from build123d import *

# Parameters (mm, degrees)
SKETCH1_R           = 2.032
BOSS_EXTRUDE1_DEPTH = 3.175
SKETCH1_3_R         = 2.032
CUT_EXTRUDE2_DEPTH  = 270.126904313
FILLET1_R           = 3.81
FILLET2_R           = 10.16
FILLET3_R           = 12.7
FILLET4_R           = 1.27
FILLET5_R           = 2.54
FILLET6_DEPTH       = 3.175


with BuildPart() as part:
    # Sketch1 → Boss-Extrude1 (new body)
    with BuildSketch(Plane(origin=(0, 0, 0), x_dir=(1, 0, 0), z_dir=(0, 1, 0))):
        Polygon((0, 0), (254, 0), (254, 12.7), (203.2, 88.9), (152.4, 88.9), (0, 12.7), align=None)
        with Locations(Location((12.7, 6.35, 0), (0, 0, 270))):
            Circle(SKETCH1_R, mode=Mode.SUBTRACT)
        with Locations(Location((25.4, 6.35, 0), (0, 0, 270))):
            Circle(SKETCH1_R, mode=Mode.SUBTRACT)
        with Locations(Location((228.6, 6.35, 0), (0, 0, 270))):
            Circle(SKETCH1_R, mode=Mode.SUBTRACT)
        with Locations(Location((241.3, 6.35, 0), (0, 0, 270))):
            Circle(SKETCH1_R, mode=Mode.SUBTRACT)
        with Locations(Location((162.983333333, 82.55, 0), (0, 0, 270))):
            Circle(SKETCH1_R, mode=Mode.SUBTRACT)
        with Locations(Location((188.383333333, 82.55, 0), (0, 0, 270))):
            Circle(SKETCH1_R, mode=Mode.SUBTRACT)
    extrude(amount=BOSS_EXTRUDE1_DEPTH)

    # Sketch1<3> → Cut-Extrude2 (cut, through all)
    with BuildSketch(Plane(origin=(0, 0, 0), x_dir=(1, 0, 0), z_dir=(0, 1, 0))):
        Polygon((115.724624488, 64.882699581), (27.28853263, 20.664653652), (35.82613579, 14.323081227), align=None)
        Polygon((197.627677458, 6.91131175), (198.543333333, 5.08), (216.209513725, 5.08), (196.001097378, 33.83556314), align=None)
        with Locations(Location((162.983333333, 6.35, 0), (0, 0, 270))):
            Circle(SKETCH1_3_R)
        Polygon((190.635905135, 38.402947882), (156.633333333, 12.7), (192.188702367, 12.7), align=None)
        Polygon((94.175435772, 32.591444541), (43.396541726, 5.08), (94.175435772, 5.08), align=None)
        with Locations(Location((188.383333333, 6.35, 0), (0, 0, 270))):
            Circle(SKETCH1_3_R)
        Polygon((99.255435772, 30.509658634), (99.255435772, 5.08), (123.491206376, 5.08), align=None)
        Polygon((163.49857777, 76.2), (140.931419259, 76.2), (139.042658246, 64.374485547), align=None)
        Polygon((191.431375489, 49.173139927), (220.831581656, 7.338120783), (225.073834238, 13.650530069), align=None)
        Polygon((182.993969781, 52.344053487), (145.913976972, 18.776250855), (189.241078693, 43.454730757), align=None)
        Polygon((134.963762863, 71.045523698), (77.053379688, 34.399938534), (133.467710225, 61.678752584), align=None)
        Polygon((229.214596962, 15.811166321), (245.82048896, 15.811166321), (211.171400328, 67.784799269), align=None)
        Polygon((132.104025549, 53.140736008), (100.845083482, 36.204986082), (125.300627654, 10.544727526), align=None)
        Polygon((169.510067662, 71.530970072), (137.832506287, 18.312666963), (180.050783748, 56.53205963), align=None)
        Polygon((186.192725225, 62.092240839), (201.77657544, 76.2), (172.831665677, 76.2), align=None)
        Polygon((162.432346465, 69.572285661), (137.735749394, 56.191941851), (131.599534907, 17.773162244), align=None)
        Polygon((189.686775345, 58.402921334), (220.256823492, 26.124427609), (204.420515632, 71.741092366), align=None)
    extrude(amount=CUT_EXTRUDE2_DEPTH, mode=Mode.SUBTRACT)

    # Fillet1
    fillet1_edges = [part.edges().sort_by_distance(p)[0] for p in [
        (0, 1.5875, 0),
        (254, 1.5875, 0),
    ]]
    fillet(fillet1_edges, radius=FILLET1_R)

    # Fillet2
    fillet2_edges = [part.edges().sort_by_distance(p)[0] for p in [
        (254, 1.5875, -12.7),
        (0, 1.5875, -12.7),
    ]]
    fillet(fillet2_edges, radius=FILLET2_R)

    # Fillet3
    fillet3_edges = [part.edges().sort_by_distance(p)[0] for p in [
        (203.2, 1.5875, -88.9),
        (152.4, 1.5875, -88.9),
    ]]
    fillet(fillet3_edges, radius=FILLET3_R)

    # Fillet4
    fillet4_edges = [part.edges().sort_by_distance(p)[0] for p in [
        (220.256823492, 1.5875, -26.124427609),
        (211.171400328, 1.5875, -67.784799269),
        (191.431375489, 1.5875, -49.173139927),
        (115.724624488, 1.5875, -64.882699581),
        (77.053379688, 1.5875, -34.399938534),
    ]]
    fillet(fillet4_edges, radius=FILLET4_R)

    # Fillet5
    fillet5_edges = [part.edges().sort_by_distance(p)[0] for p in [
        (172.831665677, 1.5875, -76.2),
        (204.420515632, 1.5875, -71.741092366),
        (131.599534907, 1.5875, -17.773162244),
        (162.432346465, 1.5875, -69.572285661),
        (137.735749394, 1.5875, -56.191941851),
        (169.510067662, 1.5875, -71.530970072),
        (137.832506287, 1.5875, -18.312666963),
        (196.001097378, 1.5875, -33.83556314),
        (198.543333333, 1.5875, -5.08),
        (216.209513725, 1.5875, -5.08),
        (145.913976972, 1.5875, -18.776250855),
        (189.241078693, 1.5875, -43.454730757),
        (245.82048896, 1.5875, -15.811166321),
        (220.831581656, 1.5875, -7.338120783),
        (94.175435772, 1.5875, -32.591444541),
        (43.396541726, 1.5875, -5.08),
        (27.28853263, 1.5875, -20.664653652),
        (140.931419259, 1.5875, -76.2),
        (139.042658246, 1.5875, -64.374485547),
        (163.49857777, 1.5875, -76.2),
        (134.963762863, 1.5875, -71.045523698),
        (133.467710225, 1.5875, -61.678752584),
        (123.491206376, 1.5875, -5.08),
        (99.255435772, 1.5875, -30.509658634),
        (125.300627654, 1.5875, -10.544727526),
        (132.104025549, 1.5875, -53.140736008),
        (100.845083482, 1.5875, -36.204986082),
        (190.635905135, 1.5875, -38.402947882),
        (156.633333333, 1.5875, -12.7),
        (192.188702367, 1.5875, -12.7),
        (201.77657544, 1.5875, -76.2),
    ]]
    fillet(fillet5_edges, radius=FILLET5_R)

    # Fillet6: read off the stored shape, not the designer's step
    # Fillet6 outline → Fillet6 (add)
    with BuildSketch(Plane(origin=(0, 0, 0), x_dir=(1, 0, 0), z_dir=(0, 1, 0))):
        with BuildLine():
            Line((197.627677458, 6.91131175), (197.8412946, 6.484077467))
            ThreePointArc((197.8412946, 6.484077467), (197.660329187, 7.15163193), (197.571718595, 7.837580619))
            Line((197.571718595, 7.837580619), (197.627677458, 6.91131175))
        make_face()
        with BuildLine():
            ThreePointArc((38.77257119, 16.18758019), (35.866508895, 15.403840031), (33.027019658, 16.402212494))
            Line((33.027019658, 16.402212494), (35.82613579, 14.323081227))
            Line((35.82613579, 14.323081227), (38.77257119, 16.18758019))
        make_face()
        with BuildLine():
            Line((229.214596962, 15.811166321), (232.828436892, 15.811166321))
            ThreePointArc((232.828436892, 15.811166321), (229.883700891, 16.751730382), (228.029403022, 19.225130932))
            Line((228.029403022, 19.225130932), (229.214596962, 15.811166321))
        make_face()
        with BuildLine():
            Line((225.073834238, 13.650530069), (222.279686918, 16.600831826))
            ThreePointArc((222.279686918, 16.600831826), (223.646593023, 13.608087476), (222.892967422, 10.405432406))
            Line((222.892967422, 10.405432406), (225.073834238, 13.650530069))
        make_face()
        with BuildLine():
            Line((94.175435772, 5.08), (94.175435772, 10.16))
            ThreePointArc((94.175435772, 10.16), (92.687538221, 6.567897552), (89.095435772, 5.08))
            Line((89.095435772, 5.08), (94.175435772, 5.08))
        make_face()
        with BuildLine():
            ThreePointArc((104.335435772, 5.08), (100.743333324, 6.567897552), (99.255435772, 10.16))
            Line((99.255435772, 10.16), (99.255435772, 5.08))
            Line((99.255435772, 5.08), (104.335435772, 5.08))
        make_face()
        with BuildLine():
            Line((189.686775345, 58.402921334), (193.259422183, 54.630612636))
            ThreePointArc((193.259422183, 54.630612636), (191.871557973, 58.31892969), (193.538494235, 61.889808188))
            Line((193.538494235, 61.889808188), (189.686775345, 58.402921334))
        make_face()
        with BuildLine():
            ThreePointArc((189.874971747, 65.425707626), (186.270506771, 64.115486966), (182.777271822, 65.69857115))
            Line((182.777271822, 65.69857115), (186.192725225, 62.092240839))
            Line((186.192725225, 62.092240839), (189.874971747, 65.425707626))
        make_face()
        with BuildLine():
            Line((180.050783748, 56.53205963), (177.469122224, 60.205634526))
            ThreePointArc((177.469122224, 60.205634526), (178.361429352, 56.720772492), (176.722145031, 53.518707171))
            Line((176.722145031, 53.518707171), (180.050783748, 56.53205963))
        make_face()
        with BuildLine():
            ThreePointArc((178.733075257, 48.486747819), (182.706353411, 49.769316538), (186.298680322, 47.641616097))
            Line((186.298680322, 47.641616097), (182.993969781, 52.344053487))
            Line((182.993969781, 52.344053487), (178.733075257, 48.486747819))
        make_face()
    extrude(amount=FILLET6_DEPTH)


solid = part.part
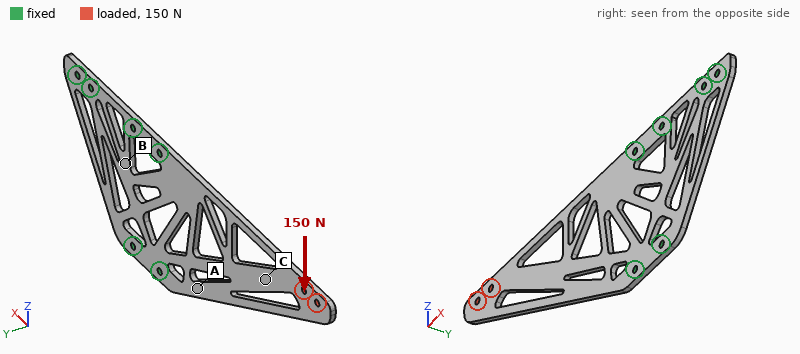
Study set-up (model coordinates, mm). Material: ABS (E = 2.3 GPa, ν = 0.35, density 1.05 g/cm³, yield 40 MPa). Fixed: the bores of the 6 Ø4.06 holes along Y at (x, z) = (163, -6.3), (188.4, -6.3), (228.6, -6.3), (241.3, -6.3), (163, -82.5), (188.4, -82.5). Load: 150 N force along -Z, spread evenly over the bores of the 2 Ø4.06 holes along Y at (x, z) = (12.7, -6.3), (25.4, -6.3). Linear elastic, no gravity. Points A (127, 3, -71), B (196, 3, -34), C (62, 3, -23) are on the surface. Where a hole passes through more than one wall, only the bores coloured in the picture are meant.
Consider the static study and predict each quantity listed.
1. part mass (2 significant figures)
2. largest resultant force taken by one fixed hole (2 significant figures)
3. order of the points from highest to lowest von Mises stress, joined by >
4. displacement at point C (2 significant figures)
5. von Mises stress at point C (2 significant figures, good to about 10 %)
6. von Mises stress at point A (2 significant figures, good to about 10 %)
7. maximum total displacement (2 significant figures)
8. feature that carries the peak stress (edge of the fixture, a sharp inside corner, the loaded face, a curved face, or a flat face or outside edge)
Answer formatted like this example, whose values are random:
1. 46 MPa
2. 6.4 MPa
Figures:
1. 32 g
2. 280 N
3. A > C > B
4. 0.91 mm
5. 3.6 MPa
6. 7.2 MPa
7. 2.3 mm
8. a curved face
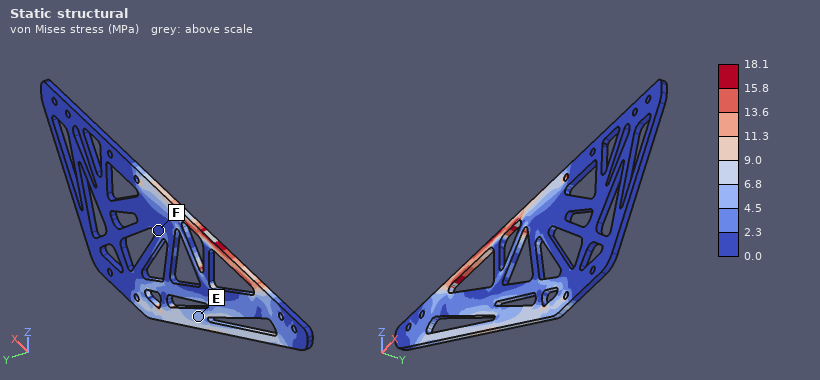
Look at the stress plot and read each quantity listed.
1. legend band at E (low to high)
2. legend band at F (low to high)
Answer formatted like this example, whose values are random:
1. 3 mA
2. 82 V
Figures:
1. 4.5 to 6.8 MPa
2. 0.0 to 2.3 MPa
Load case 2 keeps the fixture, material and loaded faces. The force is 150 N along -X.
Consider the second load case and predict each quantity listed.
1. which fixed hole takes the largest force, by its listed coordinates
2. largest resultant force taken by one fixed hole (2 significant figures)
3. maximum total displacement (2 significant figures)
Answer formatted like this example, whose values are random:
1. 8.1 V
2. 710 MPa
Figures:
1. (163, -6.3)
2. 140 N
3. 0.79 mm
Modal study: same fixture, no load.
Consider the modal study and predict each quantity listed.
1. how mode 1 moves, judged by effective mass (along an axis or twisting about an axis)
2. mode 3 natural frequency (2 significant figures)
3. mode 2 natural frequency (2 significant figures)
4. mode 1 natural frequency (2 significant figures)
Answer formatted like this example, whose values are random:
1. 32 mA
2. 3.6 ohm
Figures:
1. along Y
2. 260 Hz
3. 170 Hz
4. 36 Hz
